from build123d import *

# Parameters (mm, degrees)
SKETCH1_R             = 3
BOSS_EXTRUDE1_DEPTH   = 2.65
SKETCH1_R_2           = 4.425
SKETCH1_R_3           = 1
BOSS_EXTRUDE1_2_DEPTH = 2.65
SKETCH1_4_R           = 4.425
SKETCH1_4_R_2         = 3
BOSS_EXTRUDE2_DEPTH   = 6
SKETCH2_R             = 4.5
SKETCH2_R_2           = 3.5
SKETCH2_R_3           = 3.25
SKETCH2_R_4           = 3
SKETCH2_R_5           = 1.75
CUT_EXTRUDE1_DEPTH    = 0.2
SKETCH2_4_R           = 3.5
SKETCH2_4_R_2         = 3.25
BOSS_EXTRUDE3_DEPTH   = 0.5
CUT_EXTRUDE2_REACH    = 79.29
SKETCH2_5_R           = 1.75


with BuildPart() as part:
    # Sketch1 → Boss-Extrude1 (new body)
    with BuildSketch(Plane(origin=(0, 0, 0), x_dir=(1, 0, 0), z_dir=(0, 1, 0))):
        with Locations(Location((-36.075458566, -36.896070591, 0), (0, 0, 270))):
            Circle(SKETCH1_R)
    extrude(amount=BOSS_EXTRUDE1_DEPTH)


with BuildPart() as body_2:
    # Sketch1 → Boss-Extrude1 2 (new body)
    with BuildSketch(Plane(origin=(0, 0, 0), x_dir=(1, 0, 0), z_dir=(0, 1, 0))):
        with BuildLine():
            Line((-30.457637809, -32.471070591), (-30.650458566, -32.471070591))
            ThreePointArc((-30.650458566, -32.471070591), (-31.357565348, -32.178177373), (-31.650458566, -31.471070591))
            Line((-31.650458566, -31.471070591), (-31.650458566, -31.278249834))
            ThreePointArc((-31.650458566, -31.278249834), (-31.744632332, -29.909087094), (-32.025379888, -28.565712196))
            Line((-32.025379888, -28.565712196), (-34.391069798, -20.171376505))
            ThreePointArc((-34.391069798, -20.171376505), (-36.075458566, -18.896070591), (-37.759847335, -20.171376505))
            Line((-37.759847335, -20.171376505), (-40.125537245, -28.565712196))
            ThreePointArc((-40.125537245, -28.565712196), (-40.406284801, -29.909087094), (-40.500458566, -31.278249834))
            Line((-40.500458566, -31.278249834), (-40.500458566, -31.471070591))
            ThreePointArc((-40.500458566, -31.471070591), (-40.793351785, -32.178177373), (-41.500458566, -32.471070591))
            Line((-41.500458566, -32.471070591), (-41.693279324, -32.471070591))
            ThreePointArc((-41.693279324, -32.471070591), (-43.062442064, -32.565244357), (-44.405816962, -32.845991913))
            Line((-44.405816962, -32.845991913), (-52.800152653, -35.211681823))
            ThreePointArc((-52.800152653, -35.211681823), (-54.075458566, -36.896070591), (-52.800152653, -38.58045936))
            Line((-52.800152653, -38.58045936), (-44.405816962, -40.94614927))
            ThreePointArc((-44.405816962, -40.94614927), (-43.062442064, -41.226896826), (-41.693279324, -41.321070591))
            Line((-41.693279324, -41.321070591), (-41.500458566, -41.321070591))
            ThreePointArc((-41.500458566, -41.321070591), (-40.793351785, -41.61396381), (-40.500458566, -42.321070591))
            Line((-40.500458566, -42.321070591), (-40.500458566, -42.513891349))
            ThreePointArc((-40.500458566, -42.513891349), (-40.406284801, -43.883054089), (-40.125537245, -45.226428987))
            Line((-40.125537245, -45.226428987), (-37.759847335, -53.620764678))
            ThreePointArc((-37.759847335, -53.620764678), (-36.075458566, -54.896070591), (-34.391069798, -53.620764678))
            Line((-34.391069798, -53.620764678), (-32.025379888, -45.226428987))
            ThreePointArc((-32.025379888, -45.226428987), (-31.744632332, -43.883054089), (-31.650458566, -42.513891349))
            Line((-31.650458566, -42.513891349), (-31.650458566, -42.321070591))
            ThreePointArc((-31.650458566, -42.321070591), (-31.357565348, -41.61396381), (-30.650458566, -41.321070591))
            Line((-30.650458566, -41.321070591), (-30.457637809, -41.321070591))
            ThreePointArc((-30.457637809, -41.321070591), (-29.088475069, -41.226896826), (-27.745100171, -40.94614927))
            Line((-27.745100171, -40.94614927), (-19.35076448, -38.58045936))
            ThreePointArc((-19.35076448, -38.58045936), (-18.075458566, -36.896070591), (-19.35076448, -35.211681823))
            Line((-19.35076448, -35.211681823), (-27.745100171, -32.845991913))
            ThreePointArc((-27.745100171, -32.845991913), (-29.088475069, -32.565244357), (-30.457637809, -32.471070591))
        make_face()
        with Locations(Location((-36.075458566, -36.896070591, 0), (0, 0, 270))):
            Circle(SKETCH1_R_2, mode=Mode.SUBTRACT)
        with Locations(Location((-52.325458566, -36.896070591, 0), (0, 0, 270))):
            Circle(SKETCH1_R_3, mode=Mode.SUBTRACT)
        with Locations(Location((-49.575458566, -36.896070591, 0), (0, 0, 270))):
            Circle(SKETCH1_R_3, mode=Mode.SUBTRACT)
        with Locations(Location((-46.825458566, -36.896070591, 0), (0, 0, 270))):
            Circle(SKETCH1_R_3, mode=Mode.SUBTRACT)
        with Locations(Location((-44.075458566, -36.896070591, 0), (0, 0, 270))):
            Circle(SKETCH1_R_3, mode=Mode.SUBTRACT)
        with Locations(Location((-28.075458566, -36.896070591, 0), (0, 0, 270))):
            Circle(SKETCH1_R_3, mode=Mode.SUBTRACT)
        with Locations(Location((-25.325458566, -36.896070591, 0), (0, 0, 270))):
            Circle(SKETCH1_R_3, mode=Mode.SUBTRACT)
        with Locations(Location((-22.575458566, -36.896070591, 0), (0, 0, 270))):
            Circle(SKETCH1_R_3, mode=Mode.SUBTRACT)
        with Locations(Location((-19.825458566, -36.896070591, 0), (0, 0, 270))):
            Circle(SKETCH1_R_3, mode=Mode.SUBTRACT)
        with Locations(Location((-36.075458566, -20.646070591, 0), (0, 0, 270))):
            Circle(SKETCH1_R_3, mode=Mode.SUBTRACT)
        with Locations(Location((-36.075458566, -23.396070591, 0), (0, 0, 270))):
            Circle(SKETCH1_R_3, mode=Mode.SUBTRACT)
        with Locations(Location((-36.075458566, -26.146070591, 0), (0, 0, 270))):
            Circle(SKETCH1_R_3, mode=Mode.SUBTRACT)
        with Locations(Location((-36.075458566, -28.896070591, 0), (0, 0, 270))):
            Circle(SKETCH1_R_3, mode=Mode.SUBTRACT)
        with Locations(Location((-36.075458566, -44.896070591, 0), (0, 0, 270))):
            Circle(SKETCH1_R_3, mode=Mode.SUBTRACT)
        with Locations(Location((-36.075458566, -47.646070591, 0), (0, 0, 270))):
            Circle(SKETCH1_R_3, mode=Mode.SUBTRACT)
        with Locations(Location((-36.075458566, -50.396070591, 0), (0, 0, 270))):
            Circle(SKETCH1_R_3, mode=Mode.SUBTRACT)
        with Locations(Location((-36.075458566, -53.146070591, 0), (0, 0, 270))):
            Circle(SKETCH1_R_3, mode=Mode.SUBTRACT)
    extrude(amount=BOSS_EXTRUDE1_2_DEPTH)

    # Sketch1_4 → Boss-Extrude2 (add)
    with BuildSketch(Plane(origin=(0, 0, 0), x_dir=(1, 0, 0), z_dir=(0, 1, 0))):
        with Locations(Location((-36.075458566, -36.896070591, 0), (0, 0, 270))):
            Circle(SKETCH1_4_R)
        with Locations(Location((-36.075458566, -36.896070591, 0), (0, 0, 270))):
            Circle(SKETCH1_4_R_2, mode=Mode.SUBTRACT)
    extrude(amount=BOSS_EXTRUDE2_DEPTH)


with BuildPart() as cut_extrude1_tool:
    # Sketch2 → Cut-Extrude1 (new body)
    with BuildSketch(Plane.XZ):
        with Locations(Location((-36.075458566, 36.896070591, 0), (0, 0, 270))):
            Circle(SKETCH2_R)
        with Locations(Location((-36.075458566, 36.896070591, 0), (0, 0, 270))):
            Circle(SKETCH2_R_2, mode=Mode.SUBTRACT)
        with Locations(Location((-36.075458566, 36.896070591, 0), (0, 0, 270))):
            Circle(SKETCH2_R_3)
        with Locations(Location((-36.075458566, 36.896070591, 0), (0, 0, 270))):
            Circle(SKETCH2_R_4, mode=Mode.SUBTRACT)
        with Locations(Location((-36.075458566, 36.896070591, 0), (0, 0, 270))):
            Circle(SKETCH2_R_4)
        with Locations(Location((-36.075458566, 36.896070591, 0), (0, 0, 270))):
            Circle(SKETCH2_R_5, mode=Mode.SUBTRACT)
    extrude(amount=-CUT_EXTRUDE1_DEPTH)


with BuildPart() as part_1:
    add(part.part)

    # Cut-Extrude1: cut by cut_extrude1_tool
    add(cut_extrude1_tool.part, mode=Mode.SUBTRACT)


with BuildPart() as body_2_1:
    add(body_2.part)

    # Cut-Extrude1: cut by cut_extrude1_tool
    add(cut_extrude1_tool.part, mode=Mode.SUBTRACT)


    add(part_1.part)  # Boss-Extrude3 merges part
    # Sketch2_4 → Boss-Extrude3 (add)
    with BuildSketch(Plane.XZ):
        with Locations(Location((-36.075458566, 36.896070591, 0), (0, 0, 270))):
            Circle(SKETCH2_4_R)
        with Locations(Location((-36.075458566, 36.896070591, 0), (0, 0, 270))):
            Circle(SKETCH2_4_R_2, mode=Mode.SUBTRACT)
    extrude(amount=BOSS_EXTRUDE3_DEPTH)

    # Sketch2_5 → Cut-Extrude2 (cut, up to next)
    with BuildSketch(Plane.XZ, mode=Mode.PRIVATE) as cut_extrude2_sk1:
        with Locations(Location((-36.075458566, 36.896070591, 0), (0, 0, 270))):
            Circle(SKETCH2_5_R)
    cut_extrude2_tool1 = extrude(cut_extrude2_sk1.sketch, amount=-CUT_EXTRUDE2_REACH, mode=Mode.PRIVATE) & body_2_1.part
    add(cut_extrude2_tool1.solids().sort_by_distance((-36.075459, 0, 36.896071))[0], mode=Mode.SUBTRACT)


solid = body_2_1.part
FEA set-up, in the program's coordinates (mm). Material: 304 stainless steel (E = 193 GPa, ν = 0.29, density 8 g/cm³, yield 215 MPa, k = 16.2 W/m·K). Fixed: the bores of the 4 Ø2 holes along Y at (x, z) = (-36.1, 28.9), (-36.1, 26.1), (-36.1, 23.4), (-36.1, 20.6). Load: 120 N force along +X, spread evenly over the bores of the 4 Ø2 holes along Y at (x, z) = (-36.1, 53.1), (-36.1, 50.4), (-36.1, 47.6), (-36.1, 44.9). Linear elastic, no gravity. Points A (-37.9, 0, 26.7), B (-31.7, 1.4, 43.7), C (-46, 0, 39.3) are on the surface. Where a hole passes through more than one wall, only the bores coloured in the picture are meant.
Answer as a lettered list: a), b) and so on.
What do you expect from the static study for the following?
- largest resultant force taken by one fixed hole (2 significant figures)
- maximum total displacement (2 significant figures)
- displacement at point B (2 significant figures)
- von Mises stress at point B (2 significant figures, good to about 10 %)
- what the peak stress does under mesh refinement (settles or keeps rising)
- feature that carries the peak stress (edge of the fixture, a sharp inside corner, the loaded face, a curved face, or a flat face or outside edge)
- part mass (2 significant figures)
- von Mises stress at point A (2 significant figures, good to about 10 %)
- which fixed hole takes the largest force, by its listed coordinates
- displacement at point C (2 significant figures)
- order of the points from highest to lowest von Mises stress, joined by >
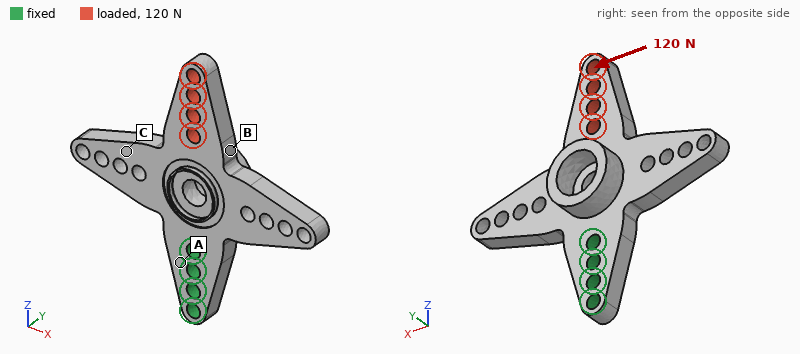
a) 450 N
b) 25 µm
c) 13 µm
d) 22 MPa
e) keeps rising
f) edge of the fixture
g) 8.5 g
h) 38 MPa
i) (-36.1, 28.9)
j) 12 µm
k) A > B > C
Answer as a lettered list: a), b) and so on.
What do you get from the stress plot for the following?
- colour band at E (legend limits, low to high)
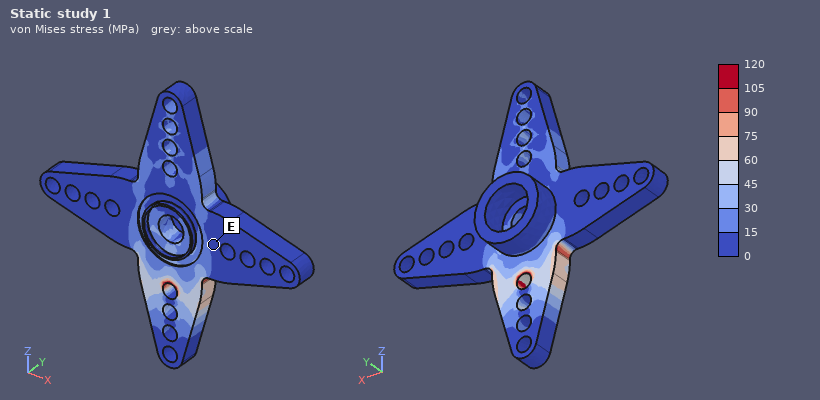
a) 0 to 15 MPa
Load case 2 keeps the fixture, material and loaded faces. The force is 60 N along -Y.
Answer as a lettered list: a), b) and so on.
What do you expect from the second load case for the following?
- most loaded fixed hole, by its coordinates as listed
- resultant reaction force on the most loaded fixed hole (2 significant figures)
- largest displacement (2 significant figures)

a) (-36.1, 28.9)
b) 160 N
c) 76 µm
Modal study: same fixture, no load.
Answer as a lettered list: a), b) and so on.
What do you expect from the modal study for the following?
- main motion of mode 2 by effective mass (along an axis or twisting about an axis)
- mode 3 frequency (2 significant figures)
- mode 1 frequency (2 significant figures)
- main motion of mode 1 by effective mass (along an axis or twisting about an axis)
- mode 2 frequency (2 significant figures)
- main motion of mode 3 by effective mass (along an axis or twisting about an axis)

a) twisting about Z
b) 7900 Hz
c) 4300 Hz
d) along Y
e) 6400 Hz
f) along X
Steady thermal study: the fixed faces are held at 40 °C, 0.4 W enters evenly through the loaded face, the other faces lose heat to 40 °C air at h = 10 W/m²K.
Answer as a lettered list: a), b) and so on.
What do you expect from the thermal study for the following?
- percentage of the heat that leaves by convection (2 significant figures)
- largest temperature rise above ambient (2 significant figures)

a) 22 %
b) 21 K
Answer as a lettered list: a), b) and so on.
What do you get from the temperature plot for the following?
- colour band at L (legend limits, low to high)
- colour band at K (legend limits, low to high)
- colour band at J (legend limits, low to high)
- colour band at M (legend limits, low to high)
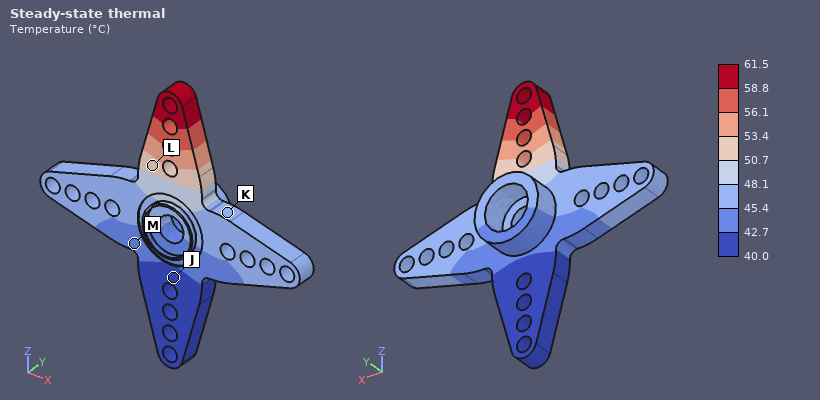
a) 50.7 to 53.4 °C
b) 45.4 to 48.1 °C
c) 40.0 to 42.7 °C
d) 42.7 to 45.4 °C
